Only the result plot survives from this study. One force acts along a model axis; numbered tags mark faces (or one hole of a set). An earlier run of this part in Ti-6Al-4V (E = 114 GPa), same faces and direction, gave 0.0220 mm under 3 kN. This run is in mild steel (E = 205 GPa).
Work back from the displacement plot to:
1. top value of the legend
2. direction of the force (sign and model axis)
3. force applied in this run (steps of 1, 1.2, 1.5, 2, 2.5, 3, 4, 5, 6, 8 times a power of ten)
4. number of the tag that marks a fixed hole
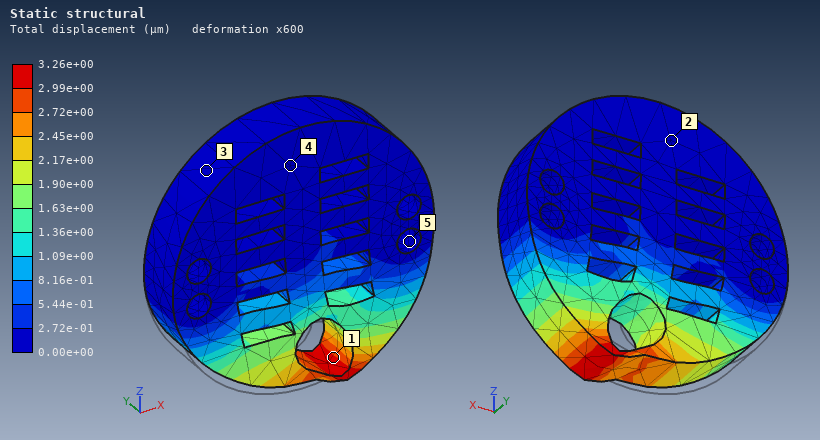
3.26e+00 µm
+X
800 N
5
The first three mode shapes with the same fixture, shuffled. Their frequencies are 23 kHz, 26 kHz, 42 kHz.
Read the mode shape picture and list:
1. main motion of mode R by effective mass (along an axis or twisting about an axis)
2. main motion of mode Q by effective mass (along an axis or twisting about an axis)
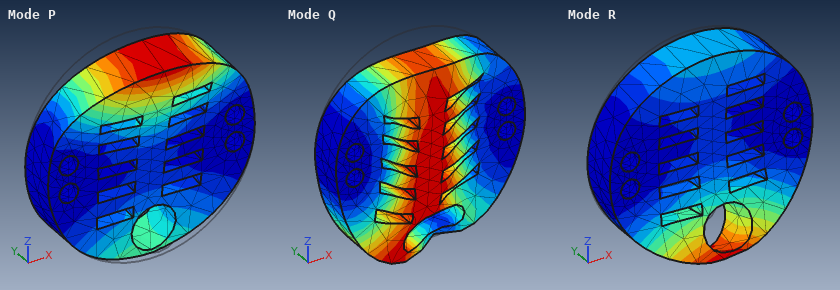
along Y
along Z
